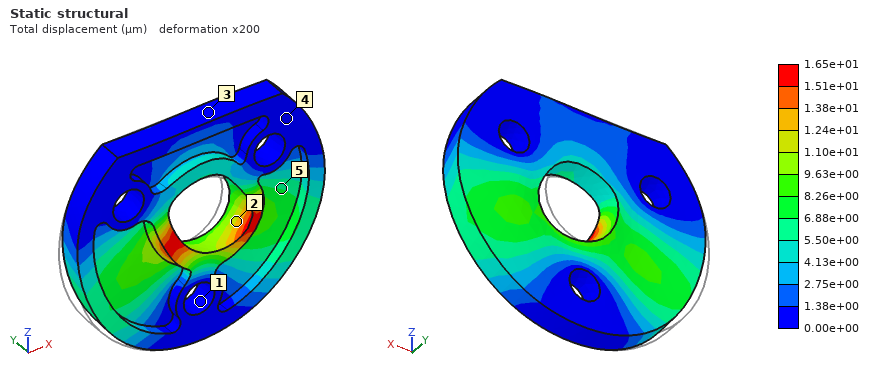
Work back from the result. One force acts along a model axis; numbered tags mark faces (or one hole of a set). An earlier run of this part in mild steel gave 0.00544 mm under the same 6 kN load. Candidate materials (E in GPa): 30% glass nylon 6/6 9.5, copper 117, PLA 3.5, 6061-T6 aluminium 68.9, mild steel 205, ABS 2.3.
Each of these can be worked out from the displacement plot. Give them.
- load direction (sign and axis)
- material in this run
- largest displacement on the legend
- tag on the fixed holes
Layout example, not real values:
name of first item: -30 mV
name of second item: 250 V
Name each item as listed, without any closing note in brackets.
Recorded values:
load direction: +X
material in this run: 6061-T6 aluminium
largest displacement on the legend: 1.65e+01 µm
tag on the fixed holes: 1
